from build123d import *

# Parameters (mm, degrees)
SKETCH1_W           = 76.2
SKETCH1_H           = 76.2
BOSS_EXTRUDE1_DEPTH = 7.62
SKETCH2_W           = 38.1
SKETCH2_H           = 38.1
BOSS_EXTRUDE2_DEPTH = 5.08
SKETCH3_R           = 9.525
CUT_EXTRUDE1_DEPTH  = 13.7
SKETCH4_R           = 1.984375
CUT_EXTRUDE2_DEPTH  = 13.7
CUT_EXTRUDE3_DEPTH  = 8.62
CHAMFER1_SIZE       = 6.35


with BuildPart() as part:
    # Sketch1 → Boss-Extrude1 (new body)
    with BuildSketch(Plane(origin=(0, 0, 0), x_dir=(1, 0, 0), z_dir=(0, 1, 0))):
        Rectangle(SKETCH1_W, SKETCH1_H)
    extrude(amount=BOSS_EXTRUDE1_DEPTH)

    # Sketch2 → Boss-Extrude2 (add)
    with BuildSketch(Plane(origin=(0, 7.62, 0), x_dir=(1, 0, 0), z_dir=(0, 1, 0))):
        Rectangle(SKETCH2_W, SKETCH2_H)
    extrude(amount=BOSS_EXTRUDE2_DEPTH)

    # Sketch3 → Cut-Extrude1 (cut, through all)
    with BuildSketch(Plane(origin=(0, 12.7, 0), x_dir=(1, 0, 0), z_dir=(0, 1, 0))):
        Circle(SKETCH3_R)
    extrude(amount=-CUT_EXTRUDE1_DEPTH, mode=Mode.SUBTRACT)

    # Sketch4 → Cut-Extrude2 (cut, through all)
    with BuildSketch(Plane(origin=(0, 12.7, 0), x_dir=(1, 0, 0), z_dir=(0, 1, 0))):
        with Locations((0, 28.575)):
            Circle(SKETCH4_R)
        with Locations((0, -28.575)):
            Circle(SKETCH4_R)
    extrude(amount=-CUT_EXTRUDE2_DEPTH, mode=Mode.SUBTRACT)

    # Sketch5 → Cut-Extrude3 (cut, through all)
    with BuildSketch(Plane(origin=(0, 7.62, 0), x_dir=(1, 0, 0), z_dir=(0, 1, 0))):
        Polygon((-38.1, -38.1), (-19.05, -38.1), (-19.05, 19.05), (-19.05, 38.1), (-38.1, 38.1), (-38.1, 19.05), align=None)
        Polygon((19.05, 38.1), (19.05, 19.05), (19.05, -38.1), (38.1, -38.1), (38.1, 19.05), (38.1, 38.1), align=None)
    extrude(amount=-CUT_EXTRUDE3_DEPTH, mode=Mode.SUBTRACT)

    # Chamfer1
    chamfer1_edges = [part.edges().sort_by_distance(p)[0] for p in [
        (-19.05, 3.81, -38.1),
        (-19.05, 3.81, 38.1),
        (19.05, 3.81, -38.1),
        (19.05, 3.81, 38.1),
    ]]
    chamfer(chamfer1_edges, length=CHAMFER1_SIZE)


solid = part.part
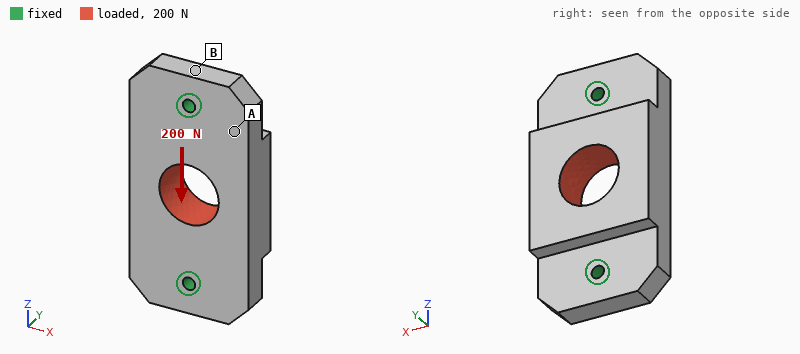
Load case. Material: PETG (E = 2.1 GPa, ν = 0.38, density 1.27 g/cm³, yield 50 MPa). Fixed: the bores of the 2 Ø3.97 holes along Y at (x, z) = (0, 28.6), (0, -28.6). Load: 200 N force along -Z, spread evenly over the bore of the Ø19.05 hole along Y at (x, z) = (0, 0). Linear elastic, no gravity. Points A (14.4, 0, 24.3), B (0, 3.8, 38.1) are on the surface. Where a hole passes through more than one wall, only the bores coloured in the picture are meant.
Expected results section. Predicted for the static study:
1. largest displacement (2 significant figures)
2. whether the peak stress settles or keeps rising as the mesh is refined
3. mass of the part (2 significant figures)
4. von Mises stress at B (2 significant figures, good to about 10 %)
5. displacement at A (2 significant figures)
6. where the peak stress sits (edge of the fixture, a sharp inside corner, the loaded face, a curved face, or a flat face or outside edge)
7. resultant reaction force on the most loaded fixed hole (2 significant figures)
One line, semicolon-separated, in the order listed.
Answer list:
7.7 µm; keeps rising; 32 g; 0.59 MPa; 4.9 µm; edge of the fixture; 100 N
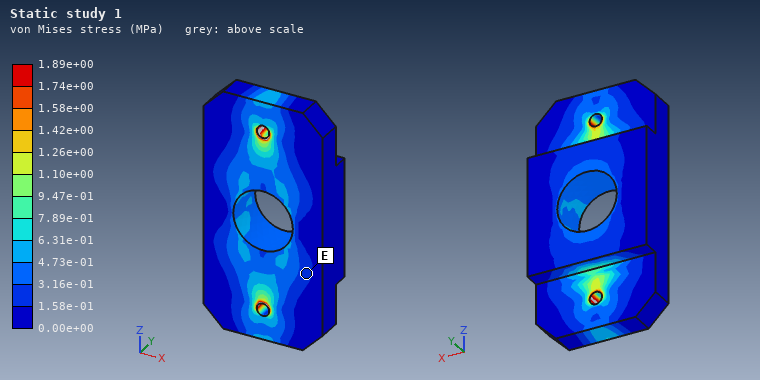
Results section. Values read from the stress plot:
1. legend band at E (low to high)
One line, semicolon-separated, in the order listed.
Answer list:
1.58e-01 to 3.16e-01 MPa
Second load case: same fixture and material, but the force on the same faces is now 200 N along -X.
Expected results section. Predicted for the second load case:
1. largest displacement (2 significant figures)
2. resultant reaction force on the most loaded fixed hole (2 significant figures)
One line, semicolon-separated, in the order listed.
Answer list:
37 µm; 100 N
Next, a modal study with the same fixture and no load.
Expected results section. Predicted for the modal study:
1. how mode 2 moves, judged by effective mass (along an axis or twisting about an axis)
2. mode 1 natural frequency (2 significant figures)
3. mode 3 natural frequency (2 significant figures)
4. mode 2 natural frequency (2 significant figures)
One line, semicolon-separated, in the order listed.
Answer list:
along Y; 1700 Hz; 4000 Hz; 2300 Hz
